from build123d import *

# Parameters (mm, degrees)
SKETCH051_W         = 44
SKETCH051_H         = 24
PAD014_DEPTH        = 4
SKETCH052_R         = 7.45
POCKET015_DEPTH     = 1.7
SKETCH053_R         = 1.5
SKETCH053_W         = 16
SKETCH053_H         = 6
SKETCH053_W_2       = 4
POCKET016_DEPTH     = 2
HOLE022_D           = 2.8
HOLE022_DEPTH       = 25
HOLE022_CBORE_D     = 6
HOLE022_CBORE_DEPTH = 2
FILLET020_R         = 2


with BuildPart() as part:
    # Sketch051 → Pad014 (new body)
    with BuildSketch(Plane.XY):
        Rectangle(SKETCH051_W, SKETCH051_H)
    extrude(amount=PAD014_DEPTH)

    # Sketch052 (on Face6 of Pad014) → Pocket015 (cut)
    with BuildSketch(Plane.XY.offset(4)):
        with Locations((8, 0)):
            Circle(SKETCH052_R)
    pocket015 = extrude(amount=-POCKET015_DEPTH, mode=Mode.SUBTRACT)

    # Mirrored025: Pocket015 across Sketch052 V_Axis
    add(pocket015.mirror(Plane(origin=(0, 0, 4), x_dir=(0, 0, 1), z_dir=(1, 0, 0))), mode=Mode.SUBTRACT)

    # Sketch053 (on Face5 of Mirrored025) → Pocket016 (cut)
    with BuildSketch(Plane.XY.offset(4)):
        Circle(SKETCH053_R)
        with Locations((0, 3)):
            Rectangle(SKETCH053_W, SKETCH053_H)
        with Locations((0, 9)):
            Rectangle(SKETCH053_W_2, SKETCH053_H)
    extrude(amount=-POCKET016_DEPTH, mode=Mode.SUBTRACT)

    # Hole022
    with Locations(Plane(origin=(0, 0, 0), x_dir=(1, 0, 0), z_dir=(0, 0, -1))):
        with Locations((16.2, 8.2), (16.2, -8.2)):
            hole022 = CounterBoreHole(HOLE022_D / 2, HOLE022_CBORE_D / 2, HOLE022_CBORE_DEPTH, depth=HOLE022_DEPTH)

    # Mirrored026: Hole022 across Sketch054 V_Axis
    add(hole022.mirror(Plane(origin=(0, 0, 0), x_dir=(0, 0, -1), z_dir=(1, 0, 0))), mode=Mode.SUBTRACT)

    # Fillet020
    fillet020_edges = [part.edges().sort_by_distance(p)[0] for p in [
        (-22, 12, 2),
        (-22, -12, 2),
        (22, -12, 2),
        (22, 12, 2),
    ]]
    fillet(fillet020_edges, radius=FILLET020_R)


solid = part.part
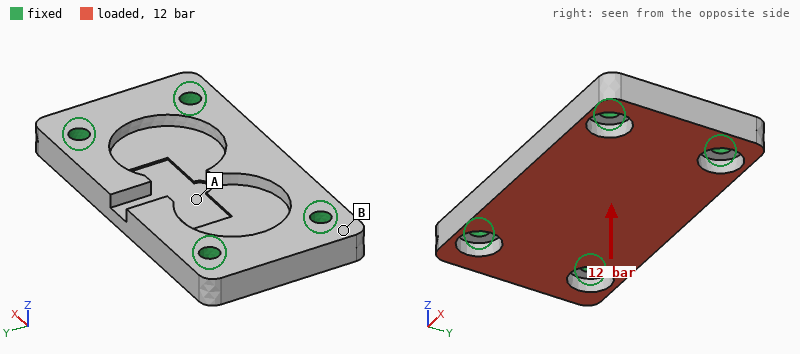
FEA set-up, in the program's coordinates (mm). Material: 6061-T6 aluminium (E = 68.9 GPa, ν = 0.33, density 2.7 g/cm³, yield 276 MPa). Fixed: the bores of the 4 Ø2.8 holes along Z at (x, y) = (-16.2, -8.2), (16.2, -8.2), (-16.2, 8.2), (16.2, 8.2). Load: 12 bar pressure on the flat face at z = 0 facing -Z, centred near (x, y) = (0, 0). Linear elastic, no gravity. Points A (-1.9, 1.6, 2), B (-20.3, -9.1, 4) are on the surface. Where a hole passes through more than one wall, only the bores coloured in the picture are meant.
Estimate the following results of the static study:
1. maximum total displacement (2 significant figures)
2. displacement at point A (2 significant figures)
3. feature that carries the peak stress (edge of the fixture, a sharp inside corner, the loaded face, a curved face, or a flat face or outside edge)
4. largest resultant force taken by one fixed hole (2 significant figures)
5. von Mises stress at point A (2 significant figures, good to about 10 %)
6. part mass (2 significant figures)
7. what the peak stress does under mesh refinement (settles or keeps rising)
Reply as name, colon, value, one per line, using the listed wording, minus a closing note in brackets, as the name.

maximum total displacement: 29 µm
displacement at point A: 28 µm
feature that carries the peak stress: edge of the fixture
largest resultant force taken by one fixed hole: 450 N
von Mises stress at point A: 21 MPa
part mass: 8.7 g
what the peak stress does under mesh refinement: keeps rising
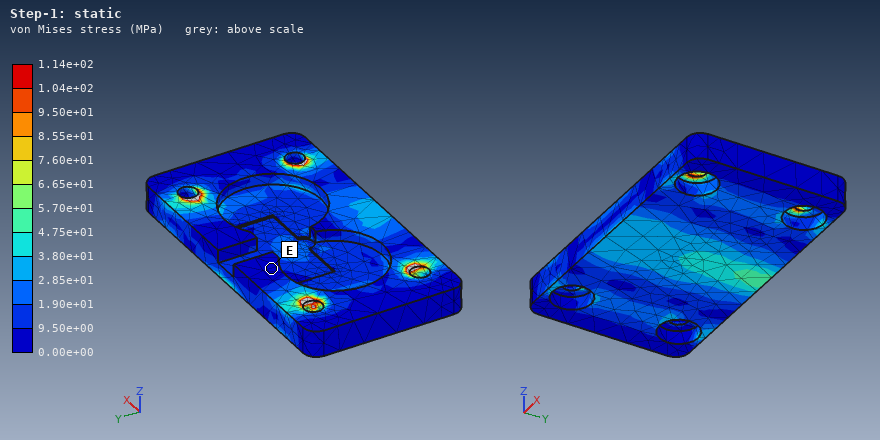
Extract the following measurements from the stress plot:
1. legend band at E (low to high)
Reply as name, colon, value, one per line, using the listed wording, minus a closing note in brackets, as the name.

legend band at E: 0.00e+00 to 9.50e+00 MPa
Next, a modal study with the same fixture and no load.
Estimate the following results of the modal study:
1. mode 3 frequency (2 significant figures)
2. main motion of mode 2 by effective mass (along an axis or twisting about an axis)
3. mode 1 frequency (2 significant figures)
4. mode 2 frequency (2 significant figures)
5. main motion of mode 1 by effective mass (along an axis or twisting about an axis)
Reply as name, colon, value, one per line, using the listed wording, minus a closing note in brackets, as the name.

mode 3 frequency: 30 kHz
main motion of mode 2 by effective mass: twisting about X
mode 1 frequency: 14 kHz
mode 2 frequency: 18 kHz
main motion of mode 1 by effective mass: along Z
